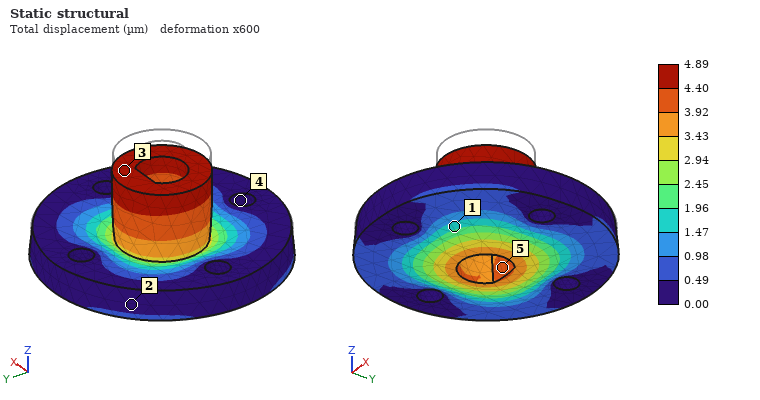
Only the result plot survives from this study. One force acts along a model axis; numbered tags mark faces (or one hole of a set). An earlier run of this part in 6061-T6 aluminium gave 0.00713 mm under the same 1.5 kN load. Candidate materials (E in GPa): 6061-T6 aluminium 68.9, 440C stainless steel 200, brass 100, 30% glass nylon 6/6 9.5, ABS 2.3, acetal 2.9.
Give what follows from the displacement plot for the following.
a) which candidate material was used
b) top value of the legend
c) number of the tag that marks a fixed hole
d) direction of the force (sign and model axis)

brass
4.89 µm
4
-Z
